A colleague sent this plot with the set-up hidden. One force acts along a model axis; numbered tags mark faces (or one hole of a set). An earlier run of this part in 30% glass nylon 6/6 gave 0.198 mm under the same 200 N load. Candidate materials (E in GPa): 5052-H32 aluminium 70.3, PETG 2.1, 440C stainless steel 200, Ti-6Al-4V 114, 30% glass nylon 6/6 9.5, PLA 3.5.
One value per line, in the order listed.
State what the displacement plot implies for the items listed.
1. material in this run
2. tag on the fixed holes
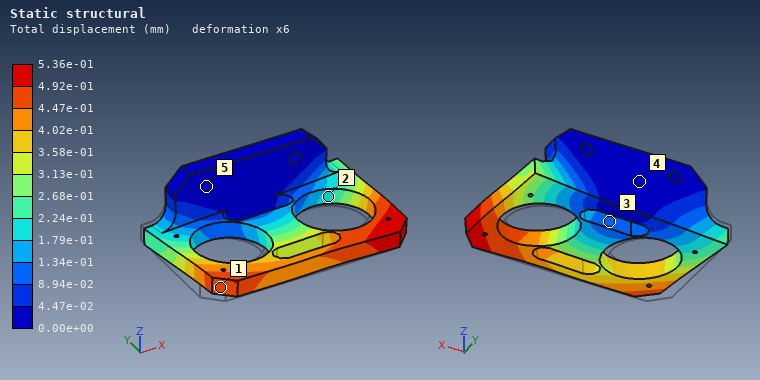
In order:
PLA
5
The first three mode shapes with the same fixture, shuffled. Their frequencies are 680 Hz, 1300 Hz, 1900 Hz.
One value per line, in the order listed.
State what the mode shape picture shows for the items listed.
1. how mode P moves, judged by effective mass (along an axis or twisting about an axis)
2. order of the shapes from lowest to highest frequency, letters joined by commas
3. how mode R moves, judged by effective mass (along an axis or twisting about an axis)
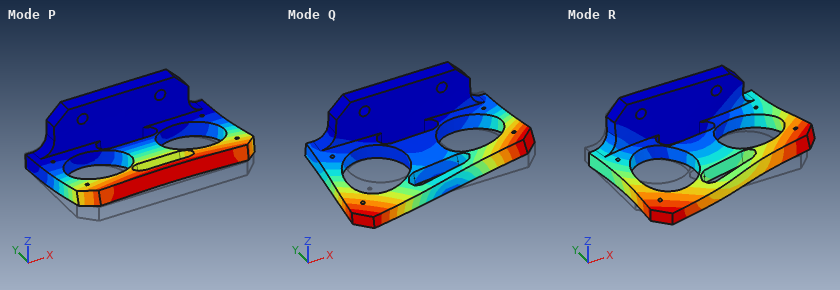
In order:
along Z
P, Q, R
along X
